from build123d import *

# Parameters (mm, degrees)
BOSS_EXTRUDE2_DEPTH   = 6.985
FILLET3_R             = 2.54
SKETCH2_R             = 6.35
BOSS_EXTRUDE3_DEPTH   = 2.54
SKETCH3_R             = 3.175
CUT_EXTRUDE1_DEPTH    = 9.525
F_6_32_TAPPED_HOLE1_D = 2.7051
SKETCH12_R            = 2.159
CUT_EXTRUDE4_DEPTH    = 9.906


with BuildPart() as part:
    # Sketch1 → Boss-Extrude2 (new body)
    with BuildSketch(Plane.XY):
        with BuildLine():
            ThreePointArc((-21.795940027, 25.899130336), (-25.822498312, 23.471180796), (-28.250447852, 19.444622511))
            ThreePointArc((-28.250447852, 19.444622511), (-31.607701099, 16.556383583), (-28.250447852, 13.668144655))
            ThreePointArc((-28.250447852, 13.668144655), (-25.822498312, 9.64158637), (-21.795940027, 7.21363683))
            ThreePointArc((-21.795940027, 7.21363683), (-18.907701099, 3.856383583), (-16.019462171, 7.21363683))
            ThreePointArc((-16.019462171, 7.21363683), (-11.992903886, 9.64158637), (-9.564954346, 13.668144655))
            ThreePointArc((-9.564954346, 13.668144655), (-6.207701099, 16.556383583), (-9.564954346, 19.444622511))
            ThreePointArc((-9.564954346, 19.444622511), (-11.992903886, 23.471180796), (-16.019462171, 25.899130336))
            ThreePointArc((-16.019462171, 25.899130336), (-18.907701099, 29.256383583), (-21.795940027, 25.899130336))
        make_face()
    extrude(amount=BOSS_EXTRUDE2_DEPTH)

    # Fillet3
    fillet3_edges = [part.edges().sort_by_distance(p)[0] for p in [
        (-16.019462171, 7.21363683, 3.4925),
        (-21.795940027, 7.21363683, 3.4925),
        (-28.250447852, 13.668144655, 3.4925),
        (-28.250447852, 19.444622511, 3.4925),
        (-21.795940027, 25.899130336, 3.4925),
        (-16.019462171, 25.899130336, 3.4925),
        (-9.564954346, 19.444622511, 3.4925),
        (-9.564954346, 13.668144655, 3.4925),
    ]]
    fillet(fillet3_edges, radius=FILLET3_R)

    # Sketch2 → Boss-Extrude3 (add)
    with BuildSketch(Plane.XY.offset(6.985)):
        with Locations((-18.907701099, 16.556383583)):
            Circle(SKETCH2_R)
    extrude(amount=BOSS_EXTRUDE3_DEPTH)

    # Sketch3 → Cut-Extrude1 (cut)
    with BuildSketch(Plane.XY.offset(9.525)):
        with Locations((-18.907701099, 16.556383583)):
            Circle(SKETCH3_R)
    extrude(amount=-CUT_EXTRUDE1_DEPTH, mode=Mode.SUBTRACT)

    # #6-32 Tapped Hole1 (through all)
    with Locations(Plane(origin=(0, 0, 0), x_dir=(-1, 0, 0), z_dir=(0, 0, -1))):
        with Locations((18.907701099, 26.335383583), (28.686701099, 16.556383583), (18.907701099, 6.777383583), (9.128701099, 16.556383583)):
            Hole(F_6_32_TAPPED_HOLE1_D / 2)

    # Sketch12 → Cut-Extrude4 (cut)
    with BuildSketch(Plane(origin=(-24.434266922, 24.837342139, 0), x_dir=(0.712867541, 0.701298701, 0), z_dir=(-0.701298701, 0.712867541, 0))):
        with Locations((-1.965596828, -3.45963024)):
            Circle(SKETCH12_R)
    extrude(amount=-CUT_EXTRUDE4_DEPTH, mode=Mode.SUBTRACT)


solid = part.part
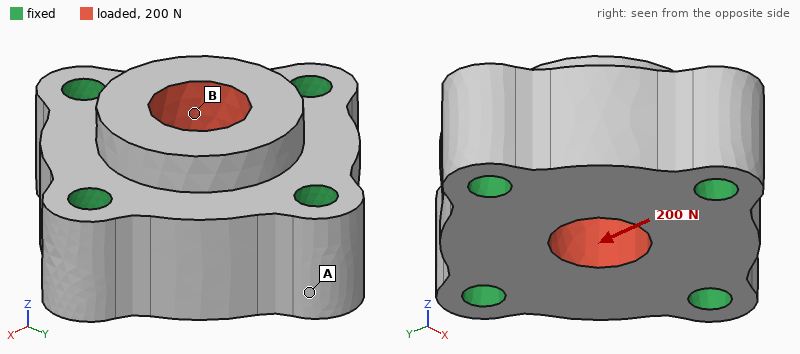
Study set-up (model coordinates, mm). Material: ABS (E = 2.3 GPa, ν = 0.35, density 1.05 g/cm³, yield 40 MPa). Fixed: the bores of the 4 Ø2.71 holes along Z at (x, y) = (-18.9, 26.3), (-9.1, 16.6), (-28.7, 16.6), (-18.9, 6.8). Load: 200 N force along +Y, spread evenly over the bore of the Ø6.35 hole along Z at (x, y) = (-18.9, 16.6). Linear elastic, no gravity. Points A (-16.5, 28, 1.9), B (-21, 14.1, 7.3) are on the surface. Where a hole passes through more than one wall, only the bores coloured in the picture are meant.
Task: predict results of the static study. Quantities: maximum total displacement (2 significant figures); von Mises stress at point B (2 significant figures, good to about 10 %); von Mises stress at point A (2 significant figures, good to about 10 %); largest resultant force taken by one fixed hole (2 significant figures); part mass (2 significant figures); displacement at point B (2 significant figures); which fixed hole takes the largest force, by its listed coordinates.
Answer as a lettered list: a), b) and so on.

a) 8.8 µm
b) 2.0 MPa
c) 0.53 MPa
d) 78 N
e) 2.4 g
f) 6.8 µm
g) (-18.9, 6.8)
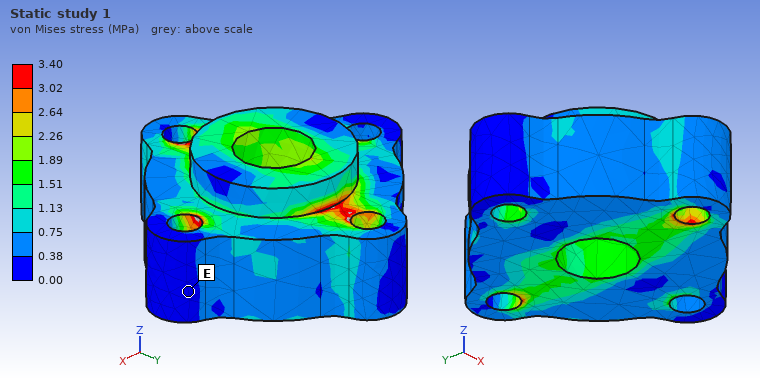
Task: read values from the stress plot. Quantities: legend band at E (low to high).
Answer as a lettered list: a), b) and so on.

a) 0.00 to 0.38 MPa
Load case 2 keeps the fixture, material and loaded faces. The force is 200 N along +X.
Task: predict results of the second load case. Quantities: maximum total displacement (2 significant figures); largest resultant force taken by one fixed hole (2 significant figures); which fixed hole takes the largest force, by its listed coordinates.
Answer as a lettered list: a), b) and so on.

a) 8.7 µm
b) 79 N
c) (-9.1, 16.6)
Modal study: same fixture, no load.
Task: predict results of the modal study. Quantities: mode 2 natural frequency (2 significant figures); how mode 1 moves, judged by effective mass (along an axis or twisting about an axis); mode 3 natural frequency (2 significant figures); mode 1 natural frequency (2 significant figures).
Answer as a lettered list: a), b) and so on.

a) 27 kHz
b) along Z
c) 28 kHz
d) 25 kHz
